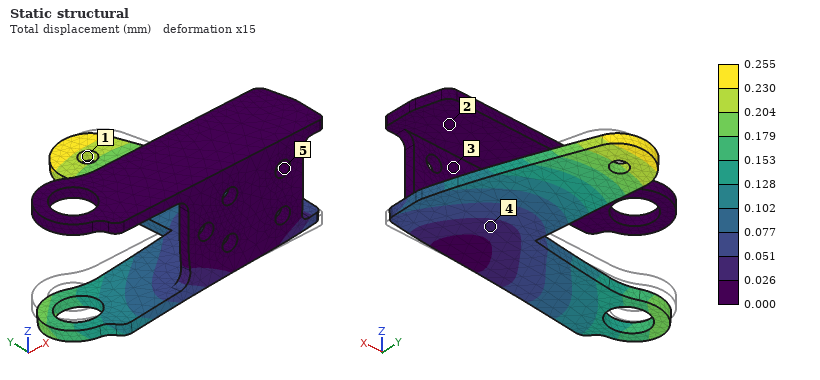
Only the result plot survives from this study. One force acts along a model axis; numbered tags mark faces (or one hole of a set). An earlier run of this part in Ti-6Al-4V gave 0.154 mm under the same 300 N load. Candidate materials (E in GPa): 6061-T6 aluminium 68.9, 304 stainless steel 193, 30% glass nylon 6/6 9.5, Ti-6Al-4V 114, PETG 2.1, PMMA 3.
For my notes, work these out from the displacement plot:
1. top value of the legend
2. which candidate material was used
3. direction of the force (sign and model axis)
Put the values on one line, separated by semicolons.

0.255 mm; 6061-T6 aluminium; -X
